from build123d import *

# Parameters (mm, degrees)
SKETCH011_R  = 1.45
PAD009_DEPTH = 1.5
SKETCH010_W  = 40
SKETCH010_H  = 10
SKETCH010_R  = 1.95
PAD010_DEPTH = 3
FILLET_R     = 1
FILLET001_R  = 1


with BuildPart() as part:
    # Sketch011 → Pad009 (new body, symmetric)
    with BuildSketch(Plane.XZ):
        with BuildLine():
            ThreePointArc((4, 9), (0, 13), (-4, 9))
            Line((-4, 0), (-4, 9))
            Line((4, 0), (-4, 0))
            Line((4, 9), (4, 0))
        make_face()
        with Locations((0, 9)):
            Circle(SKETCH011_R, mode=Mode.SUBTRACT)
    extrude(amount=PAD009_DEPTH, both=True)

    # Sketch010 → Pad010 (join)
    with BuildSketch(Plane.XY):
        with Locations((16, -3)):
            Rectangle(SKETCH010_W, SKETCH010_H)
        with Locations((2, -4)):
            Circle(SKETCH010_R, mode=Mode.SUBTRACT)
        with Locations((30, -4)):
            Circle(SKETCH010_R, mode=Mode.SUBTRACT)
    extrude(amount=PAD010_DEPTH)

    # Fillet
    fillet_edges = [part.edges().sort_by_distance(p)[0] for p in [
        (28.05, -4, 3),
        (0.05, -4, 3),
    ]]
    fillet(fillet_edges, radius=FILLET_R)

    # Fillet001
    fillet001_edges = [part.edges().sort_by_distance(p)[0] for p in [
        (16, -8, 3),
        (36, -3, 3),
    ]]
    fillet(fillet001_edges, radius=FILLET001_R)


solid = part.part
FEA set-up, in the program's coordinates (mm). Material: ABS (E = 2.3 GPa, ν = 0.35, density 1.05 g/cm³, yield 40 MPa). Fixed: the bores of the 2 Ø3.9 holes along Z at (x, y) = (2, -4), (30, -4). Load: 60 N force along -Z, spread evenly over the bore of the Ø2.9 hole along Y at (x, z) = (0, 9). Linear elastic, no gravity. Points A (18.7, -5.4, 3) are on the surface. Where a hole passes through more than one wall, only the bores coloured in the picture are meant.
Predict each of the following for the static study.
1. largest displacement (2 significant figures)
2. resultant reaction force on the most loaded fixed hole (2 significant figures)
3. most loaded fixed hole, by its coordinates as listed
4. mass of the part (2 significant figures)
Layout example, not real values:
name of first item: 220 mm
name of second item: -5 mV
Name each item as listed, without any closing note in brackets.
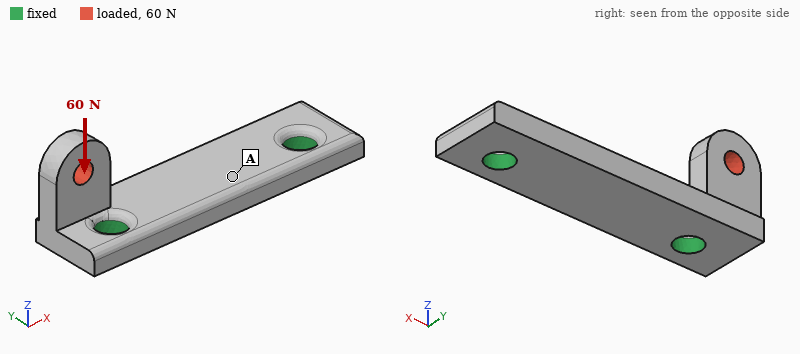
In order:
largest displacement: 0.14 mm
resultant reaction force on the most loaded fixed hole: 61 N
most loaded fixed hole, by its coordinates as listed: (2, -4)
mass of the part: 1.4 g
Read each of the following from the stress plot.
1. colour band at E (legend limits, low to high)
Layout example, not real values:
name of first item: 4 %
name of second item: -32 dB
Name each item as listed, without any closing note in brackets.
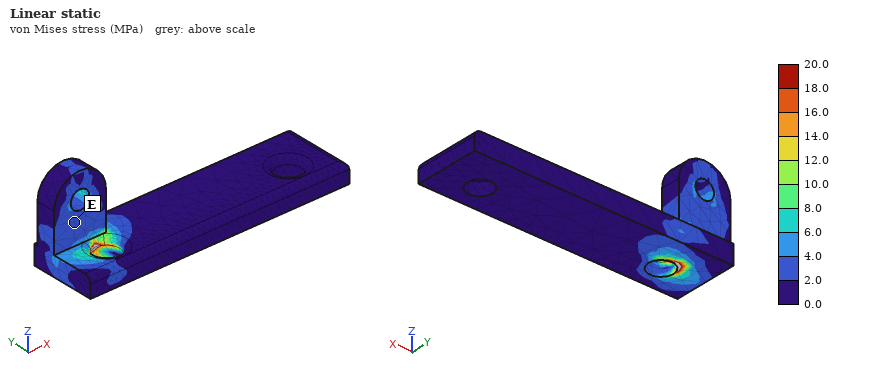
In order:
colour band at E: 2.0 to 4.0 MPa
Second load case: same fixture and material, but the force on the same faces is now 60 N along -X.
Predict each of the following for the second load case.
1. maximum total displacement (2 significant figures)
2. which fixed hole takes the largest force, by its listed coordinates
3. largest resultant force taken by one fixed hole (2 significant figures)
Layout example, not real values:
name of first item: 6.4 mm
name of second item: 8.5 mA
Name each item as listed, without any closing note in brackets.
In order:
maximum total displacement: 0.30 mm
which fixed hole takes the largest force, by its listed coordinates: (2, -4)
largest resultant force taken by one fixed hole: 46 N
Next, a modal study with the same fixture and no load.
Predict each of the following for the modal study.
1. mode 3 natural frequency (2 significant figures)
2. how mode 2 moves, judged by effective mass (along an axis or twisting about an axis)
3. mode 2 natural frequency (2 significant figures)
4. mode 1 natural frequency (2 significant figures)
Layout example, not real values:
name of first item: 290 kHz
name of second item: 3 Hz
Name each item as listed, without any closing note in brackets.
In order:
mode 3 natural frequency: 6800 Hz
how mode 2 moves, judged by effective mass: along Z
mode 2 natural frequency: 5400 Hz
mode 1 natural frequency: 4500 Hz
